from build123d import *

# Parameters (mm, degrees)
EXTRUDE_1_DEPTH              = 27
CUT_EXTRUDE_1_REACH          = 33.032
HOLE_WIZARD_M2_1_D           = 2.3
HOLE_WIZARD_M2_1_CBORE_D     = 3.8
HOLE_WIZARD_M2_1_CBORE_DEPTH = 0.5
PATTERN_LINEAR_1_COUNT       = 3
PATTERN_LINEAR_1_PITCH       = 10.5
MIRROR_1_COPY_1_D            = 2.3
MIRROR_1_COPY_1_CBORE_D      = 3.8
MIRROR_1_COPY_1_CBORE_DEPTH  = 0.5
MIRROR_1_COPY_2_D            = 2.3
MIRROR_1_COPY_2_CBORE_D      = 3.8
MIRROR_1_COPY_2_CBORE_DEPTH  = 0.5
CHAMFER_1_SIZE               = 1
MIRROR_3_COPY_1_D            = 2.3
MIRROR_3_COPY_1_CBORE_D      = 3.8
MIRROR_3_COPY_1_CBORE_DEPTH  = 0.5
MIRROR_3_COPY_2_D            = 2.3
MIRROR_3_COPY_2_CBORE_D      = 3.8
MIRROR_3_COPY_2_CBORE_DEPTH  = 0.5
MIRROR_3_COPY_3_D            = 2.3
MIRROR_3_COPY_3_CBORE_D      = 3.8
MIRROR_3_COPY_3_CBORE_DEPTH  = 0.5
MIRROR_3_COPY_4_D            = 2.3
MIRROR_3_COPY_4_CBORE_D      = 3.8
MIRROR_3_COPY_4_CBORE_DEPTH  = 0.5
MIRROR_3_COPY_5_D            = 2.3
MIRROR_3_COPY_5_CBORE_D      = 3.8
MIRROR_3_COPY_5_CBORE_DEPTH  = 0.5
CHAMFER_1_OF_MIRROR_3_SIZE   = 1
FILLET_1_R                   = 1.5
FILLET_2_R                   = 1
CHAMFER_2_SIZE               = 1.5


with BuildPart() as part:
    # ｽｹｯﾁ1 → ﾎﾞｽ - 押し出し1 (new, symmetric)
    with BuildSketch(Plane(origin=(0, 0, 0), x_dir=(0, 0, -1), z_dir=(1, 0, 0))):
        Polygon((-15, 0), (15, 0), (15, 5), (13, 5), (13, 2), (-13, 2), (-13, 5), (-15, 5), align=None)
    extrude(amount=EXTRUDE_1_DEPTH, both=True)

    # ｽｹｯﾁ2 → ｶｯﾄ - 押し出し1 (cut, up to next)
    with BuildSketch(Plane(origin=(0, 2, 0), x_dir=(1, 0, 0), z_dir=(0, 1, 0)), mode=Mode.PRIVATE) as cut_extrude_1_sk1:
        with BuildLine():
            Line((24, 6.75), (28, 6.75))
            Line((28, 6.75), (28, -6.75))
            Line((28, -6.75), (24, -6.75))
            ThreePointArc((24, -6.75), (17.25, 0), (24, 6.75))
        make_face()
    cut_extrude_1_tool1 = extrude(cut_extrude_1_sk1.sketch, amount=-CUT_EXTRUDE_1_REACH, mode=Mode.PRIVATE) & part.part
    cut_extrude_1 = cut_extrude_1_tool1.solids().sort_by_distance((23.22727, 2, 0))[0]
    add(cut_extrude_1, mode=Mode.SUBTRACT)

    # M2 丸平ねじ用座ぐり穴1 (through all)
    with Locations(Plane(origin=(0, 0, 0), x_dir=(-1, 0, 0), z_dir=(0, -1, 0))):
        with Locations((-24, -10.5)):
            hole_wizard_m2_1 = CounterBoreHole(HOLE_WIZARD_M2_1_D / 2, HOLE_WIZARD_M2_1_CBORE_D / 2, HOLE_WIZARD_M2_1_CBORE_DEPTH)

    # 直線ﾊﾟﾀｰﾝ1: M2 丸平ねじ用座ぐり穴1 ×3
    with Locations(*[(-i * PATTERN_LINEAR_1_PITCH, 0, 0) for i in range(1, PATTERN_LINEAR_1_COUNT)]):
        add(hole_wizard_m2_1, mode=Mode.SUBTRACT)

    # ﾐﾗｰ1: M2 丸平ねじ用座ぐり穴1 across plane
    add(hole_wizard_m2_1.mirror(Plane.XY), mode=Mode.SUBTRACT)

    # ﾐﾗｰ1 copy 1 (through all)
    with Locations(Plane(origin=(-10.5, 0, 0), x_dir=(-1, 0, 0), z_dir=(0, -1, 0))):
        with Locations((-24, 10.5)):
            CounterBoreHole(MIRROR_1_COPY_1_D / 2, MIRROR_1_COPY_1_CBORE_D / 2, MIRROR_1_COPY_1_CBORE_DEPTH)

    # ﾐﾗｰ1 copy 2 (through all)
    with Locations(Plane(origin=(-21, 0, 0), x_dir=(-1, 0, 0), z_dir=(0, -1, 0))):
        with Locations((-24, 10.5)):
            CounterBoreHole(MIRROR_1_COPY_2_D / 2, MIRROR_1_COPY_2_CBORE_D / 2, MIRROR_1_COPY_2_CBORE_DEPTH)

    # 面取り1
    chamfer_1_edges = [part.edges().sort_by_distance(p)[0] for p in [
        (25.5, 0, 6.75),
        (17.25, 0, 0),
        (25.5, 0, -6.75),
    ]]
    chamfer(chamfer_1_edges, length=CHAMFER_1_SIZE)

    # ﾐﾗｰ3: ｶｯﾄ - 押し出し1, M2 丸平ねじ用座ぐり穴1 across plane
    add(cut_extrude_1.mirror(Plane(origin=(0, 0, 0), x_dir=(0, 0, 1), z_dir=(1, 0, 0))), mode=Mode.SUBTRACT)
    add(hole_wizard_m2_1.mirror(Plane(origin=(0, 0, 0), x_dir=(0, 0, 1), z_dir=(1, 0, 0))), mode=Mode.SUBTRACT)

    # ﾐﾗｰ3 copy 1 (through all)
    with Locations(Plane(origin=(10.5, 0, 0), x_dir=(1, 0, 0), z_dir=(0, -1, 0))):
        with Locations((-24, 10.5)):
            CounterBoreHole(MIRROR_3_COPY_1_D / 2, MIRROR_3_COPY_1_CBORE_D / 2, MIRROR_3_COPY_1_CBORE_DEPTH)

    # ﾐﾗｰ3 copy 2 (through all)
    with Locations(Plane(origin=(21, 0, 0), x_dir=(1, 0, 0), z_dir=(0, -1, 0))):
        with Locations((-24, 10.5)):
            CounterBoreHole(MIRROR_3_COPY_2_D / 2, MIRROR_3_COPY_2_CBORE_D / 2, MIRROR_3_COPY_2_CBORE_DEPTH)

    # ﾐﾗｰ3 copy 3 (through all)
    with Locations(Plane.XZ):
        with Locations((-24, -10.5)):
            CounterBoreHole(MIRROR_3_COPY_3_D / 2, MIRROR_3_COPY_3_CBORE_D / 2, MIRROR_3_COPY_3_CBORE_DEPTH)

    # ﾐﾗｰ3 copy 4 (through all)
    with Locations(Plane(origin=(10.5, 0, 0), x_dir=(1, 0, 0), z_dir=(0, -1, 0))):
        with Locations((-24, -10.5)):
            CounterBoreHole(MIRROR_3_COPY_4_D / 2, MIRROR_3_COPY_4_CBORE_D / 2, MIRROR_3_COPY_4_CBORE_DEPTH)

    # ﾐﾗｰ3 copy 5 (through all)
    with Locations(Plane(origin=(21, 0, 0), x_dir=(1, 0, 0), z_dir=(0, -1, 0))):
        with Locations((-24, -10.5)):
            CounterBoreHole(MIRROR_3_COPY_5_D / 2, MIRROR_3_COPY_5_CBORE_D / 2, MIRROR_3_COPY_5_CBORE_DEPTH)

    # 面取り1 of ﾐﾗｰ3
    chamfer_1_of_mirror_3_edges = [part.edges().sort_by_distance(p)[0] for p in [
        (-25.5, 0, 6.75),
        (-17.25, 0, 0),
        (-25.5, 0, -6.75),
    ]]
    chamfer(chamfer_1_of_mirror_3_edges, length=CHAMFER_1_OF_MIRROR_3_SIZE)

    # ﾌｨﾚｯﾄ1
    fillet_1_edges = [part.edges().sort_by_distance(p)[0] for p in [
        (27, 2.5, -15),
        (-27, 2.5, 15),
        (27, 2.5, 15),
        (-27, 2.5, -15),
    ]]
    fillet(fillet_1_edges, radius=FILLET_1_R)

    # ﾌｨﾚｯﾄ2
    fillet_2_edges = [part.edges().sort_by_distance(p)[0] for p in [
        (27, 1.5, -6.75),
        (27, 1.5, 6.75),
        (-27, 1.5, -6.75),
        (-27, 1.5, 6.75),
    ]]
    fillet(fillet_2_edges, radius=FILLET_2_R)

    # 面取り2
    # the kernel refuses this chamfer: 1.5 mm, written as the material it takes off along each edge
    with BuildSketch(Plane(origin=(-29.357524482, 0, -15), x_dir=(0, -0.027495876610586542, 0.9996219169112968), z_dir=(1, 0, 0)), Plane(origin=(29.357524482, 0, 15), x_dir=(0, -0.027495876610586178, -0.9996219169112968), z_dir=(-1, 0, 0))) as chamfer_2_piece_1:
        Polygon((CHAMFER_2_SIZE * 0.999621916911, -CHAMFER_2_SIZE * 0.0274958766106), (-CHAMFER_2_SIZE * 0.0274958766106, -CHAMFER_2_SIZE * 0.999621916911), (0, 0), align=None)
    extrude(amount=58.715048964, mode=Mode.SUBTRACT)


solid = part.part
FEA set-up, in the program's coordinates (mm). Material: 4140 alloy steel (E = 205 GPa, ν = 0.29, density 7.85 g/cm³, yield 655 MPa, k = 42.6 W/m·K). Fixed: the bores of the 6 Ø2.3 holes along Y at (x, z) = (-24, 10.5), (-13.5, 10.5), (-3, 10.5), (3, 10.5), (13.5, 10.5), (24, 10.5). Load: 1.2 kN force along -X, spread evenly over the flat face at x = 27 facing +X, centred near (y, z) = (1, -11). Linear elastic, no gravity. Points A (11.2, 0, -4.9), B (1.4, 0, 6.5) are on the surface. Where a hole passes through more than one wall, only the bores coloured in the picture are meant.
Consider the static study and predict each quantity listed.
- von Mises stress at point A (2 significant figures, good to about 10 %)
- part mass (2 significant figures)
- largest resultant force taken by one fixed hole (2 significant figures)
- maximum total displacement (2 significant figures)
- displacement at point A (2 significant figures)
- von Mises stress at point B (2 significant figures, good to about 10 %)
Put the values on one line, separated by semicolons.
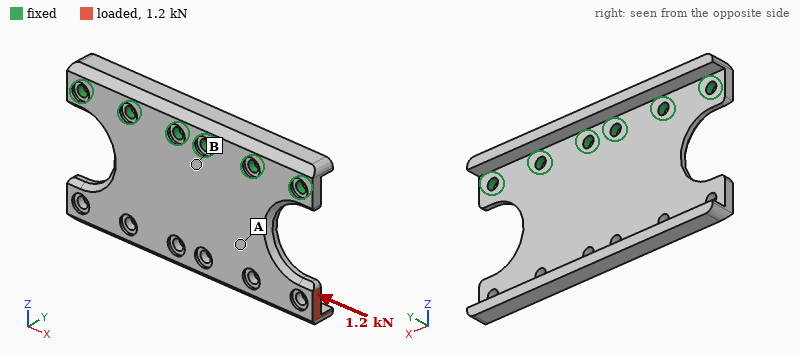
53 MPa; 25 g; 610 N; 28 µm; 8.1 µm; 21 MPa
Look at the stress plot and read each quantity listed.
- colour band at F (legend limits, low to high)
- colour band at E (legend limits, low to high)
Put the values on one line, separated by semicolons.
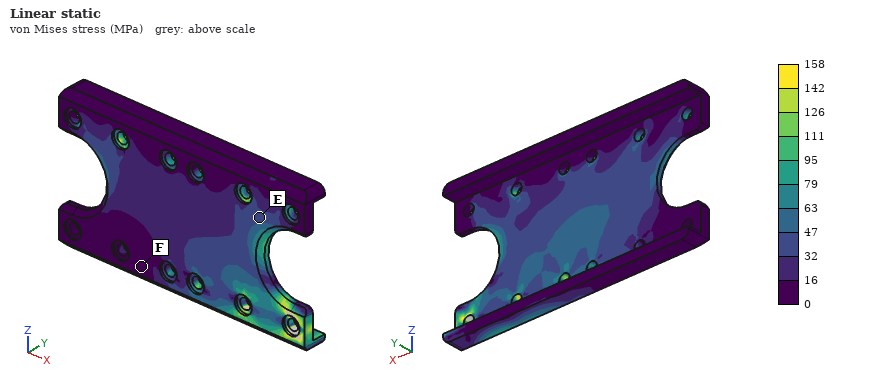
0 to 16 MPa; 32 to 47 MPa
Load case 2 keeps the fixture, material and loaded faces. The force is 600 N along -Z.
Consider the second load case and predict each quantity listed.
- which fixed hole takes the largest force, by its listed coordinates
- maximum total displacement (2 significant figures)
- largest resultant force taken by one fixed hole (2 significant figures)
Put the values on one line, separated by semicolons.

(13.5, 10.5); 57 µm; 600 N
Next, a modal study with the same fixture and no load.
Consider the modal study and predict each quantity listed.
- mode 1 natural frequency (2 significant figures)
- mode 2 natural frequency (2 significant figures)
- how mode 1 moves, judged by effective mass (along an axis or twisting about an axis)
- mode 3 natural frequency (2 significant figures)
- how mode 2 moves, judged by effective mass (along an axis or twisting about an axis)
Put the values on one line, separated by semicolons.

1900 Hz; 2700 Hz; along Y; 8400 Hz; twisting about Z
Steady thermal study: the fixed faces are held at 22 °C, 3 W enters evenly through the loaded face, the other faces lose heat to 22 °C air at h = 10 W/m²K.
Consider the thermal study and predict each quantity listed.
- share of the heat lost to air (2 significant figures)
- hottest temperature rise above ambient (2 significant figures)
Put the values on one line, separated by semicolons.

14 %; 80 K
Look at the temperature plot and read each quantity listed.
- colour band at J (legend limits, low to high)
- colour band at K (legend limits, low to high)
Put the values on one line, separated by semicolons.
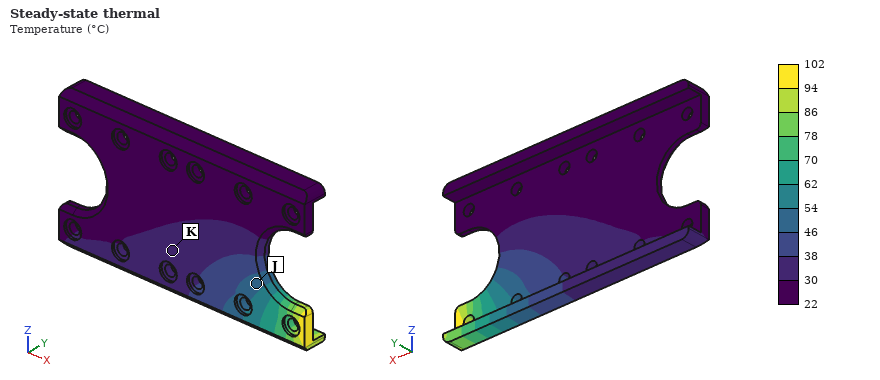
46 to 54 °C; 30 to 38 °C
